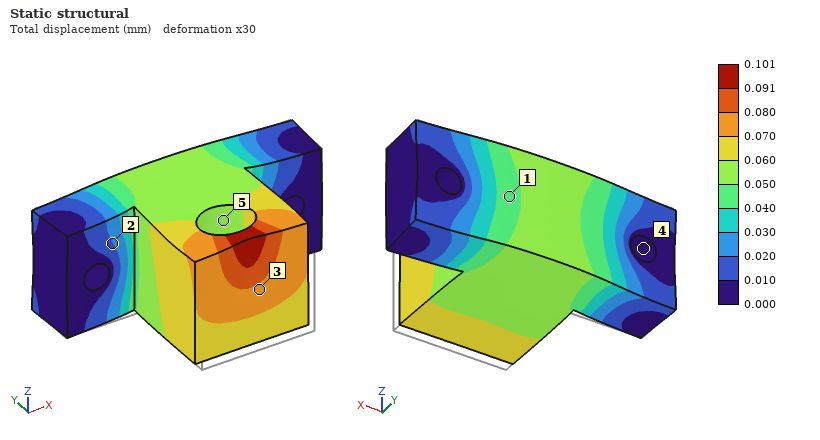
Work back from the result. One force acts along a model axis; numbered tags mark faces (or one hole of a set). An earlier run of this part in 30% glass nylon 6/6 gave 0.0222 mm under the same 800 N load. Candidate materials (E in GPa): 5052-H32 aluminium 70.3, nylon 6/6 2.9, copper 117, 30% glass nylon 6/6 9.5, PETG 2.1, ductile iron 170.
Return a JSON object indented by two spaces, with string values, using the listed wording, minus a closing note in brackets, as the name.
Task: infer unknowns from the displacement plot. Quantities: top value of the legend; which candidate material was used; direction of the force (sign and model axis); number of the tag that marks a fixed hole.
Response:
{
  "top value of the legend": "0.101 mm",
  "which candidate material was used": "PETG",
  "direction of the force": "+Y",
  "number of the tag that marks a fixed hole": "4"
}
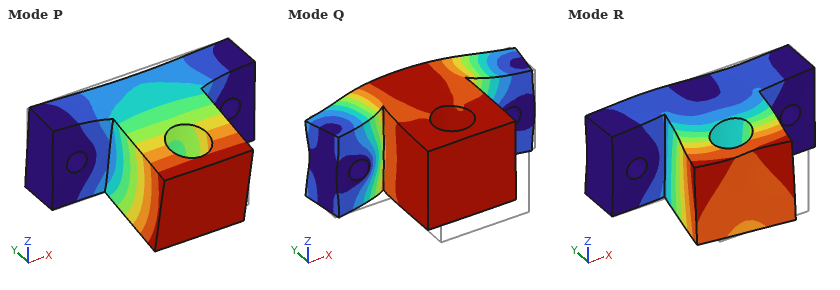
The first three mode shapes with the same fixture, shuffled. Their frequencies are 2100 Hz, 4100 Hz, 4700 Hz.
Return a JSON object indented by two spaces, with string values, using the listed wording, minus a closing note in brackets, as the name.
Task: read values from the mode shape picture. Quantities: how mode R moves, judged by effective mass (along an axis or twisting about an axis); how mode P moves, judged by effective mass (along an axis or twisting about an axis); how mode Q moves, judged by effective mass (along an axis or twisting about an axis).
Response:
{
  "how mode R moves, judged by effective mass": "along X",
  "how mode P moves, judged by effective mass": "along Z",
  "how mode Q moves, judged by effective mass": "along Y"
}
